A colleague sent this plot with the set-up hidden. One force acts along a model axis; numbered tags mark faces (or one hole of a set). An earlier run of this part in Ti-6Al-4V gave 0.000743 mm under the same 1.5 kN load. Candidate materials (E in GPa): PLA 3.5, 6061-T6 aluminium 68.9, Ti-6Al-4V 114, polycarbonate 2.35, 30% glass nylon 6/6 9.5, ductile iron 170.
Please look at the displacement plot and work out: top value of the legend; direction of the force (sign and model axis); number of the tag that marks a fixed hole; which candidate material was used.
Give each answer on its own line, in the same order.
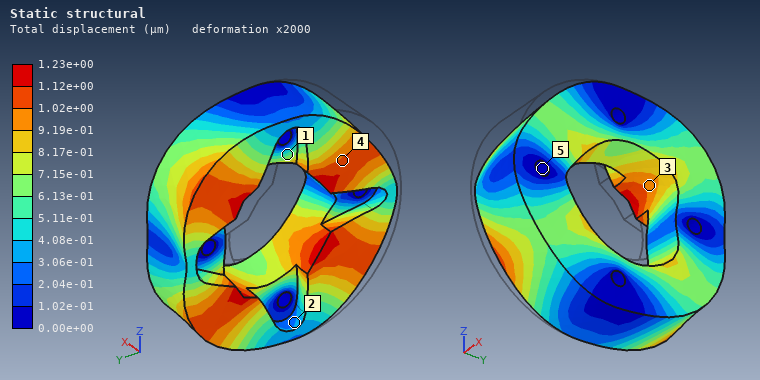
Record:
1.23e+00 µm
+Y
5
6061-T6 aluminium
